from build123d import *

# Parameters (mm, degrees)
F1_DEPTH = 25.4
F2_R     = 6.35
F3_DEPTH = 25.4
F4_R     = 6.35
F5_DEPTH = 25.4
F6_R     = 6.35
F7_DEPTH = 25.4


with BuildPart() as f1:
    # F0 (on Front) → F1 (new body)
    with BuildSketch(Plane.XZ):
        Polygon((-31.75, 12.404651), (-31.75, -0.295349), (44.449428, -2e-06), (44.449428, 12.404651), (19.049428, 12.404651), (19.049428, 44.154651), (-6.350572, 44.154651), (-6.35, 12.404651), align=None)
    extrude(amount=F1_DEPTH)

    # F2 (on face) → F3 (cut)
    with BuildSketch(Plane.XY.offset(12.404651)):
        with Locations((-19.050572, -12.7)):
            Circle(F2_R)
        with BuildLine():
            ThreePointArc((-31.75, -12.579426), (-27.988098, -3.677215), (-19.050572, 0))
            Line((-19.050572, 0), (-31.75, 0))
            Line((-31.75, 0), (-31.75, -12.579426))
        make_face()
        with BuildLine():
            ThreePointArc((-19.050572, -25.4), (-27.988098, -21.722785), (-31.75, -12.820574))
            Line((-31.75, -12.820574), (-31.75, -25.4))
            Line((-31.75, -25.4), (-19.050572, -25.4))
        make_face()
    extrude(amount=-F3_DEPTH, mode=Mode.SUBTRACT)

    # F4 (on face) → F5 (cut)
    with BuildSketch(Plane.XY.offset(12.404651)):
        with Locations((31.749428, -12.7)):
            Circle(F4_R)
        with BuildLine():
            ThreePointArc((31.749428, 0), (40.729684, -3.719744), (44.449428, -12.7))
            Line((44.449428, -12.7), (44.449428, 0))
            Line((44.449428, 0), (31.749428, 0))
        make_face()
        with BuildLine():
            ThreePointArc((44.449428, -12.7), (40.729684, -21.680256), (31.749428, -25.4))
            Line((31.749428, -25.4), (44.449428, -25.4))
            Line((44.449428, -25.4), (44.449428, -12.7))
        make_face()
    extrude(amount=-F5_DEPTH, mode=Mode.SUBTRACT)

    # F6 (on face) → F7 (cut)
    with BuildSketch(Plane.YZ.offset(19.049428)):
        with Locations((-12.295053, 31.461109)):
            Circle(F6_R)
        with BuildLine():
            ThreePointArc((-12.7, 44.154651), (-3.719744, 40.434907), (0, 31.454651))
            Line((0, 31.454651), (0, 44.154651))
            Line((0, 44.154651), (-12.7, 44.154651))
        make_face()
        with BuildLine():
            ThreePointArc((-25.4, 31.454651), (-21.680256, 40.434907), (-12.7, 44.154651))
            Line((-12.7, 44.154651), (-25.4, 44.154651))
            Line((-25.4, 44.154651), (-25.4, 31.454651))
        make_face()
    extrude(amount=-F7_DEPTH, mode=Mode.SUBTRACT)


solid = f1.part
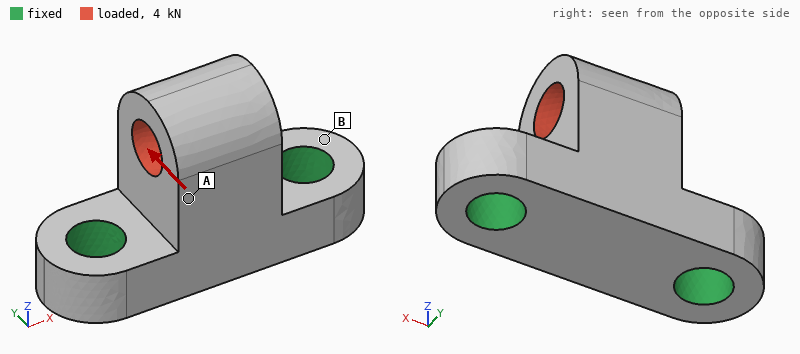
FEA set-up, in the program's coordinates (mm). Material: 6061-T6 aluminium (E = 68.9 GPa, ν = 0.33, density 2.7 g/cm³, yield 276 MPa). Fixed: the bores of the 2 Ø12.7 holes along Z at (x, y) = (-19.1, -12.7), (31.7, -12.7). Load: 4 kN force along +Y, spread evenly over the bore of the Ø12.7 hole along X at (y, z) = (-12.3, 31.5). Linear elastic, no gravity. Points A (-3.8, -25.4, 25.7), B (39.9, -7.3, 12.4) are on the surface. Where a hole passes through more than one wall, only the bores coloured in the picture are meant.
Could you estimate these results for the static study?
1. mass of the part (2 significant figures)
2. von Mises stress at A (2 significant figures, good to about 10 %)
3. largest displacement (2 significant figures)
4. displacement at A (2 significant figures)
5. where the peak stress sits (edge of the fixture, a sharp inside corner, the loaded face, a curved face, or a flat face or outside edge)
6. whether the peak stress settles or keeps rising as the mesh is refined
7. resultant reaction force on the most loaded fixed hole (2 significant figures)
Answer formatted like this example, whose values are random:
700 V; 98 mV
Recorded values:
94 g; 23 MPa; 89 µm; 52 µm; edge of the fixture; keeps rising; 2.0 kN
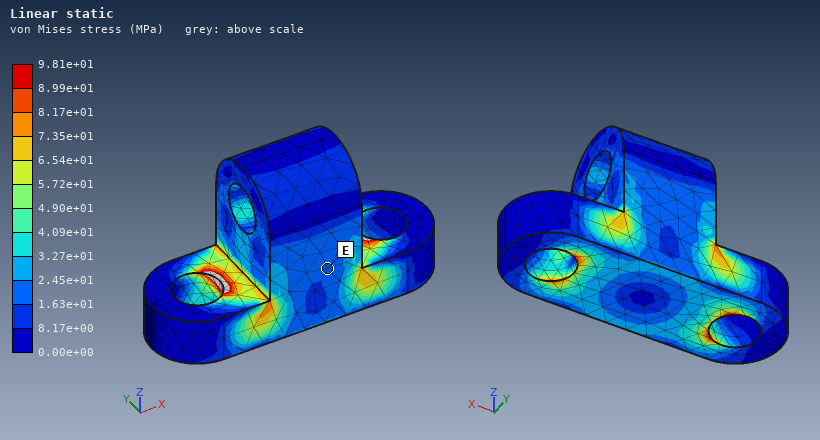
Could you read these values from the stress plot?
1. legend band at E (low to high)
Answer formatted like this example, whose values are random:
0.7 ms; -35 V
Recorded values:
1.63e+01 to 2.45e+01 MPa
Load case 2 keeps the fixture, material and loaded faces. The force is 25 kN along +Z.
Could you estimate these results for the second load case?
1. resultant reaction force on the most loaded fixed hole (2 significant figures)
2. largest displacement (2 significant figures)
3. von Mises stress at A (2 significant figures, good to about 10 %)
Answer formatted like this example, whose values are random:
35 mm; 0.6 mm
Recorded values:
13 kN; 59 µm; 30 MPa
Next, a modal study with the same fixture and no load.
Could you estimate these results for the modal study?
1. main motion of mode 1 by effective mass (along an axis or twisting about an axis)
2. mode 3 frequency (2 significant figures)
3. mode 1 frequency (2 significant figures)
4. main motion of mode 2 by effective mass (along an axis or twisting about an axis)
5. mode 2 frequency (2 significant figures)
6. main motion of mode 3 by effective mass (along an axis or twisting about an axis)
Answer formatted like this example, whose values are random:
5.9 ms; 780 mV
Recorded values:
along Y; 17 kHz; 6900 Hz; along X; 12 kHz; along Z
